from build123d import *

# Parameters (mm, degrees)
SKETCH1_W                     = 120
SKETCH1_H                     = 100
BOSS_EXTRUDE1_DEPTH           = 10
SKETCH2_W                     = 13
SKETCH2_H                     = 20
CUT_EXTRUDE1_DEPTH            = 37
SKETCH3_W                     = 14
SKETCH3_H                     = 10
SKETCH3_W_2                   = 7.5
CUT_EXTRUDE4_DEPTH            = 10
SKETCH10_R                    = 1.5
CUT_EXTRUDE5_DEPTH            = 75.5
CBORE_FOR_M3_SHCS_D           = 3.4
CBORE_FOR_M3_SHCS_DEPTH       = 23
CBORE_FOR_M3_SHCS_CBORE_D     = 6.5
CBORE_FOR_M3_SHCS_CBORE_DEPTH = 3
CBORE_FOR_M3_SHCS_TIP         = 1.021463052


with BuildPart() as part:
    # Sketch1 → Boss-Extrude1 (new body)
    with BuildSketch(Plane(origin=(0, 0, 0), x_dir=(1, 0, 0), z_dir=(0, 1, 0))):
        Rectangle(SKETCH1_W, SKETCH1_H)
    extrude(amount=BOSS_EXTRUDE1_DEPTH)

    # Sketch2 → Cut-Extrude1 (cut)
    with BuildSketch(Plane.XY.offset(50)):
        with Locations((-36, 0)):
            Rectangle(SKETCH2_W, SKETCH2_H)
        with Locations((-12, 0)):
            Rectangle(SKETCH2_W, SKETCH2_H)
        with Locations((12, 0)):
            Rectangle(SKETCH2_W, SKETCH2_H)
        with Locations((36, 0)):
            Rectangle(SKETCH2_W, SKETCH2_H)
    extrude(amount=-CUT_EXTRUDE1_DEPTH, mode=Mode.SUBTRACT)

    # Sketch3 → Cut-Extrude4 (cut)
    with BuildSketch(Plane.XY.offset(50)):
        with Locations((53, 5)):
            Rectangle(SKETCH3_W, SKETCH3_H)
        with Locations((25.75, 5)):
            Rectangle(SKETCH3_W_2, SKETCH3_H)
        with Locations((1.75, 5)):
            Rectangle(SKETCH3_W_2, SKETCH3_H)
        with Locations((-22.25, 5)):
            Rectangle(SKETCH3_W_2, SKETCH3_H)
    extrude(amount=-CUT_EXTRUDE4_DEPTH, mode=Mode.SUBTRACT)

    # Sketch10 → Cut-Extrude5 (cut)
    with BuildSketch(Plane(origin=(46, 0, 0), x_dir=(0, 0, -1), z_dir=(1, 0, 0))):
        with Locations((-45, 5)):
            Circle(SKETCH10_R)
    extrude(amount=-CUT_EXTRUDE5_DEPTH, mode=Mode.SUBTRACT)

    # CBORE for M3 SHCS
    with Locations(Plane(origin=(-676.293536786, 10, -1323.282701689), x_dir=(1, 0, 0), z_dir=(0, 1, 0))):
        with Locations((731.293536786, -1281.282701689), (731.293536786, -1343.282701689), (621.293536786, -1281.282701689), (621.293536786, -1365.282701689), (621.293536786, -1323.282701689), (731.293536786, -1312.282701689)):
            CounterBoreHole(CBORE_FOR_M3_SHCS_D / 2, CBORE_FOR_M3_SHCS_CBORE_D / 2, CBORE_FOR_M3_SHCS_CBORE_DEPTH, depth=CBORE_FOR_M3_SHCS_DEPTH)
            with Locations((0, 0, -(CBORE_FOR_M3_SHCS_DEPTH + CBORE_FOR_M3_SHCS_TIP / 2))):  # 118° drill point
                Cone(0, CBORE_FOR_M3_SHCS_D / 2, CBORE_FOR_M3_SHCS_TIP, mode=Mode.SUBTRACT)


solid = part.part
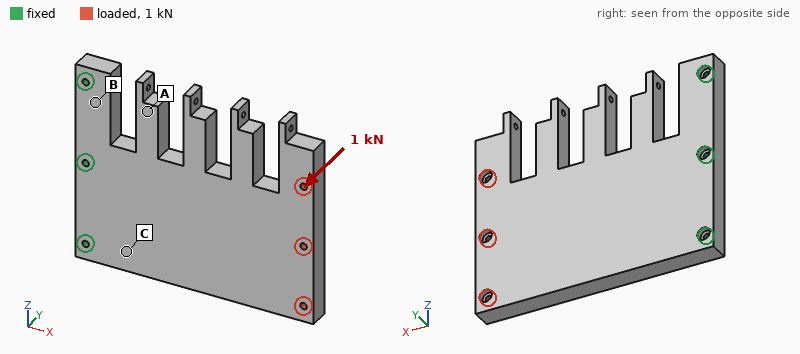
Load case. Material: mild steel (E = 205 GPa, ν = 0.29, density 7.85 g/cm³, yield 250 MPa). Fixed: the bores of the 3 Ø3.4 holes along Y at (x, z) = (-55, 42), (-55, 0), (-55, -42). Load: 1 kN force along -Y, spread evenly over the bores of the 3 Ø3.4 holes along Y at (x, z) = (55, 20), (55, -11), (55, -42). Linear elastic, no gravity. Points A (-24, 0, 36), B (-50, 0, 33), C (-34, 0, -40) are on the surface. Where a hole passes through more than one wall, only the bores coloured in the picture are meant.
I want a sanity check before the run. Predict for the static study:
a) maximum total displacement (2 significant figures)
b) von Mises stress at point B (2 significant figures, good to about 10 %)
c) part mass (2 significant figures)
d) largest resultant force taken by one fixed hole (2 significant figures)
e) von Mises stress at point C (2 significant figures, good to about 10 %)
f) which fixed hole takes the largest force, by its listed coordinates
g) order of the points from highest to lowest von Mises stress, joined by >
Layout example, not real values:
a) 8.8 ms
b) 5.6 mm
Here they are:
a) 0.65 mm
b) 53 MPa
c) 750 g
d) 930 N
e) 82 MPa
f) (-55, 0)
g) C > B > A
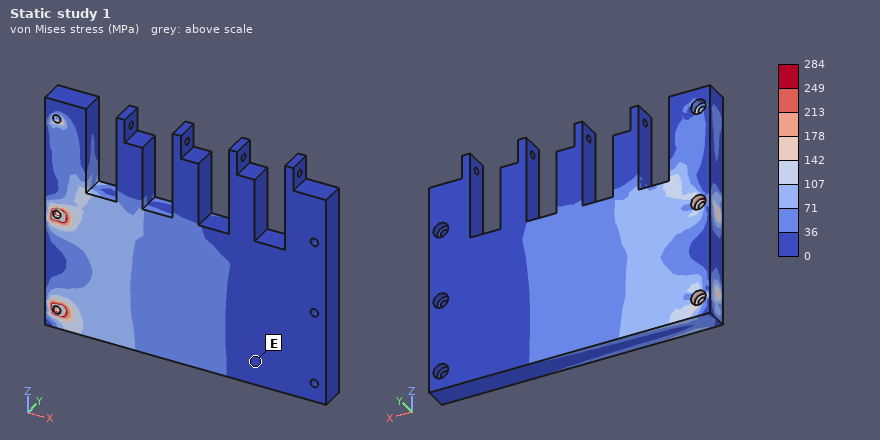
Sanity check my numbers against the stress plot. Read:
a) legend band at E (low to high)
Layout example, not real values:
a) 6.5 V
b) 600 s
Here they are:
a) 0 to 36 MPa
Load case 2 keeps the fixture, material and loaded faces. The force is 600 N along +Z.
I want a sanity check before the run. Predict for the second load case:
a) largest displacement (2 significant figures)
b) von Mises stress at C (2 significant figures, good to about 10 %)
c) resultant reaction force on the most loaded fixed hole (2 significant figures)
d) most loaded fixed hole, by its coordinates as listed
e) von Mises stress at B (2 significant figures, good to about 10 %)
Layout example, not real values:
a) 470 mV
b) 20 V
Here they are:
a) 13 µm
b) 6.9 MPa
c) 1.4 kN
d) (-55, -42)
e) 3.3 MPa
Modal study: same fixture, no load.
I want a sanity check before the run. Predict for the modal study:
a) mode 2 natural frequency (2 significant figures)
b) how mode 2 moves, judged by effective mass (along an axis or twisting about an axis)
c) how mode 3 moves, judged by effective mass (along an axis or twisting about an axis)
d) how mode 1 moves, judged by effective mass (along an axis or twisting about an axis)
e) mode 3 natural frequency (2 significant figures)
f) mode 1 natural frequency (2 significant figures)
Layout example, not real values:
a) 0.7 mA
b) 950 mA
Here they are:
a) 1400 Hz
b) twisting about X
c) along Z
d) along Y
e) 2500 Hz
f) 440 Hz
